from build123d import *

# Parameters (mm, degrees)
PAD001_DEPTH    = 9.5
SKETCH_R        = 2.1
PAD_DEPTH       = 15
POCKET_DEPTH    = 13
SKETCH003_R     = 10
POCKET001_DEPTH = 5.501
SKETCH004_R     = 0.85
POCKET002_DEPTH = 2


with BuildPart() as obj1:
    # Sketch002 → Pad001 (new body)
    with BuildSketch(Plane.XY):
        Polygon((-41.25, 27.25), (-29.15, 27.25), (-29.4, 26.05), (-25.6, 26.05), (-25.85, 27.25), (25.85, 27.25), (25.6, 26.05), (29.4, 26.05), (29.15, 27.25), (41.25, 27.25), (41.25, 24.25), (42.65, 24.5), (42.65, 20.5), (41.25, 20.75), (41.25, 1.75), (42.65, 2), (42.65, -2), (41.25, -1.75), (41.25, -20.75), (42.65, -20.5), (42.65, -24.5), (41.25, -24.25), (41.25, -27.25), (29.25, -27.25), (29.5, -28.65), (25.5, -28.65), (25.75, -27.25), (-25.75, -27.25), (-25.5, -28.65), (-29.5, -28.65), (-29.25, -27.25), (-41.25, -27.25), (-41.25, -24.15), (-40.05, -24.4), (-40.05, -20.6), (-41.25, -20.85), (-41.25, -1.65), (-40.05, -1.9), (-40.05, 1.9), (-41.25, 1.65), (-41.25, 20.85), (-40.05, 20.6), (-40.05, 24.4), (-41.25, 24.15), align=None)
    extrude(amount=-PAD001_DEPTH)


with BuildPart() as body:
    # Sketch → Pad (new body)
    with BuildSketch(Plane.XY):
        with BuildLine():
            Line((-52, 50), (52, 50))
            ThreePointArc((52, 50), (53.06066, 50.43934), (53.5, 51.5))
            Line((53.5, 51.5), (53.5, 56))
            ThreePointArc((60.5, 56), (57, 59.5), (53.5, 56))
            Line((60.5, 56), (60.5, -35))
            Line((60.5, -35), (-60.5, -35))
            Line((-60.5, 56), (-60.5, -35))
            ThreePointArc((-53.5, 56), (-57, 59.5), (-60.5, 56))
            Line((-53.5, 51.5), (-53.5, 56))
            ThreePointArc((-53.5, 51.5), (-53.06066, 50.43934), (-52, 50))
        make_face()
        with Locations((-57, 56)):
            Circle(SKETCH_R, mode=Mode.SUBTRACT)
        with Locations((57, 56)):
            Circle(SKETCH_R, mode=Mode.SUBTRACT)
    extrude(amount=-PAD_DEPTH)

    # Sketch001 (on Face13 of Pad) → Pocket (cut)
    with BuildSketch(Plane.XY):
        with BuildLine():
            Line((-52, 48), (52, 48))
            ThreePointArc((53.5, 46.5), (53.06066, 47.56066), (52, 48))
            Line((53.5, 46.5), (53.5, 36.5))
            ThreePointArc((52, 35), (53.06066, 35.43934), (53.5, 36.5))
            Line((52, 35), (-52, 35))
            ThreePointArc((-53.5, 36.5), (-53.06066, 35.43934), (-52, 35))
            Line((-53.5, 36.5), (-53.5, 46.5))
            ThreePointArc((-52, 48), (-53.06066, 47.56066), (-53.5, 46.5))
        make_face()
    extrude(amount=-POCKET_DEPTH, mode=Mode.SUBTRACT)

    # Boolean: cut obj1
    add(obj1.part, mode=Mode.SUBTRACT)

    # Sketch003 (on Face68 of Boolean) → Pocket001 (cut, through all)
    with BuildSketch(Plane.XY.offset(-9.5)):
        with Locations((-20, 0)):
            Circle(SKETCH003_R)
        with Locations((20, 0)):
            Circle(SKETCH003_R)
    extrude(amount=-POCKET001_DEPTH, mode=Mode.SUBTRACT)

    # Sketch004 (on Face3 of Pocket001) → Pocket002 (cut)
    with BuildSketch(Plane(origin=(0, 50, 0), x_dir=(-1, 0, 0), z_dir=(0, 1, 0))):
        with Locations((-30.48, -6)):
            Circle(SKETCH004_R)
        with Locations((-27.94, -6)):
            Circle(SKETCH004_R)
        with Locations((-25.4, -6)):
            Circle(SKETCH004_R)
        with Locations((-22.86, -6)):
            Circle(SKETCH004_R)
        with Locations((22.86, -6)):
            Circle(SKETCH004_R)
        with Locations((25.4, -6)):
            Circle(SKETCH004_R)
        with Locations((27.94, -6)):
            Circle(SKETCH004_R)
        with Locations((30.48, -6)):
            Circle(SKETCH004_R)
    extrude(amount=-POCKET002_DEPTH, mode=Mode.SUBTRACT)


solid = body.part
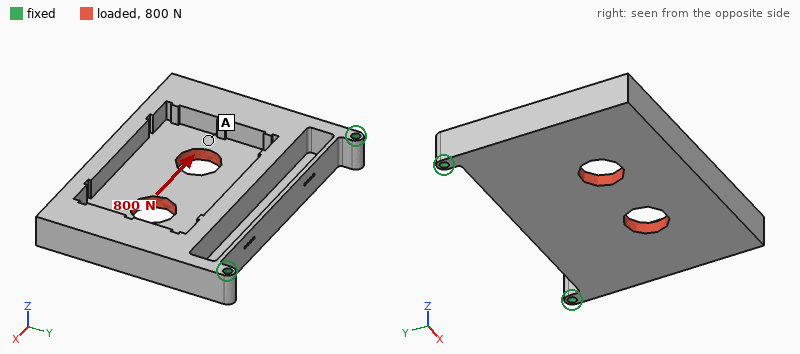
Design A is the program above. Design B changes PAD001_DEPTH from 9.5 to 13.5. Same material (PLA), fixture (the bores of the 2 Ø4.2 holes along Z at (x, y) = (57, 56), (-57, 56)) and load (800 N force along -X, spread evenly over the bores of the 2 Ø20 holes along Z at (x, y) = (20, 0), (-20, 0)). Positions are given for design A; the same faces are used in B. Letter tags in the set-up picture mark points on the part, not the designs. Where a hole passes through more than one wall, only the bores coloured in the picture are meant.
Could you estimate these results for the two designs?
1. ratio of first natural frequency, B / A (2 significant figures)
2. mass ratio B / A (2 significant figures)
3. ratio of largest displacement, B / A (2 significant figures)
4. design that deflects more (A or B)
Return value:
1.1
0.83
1.5
B
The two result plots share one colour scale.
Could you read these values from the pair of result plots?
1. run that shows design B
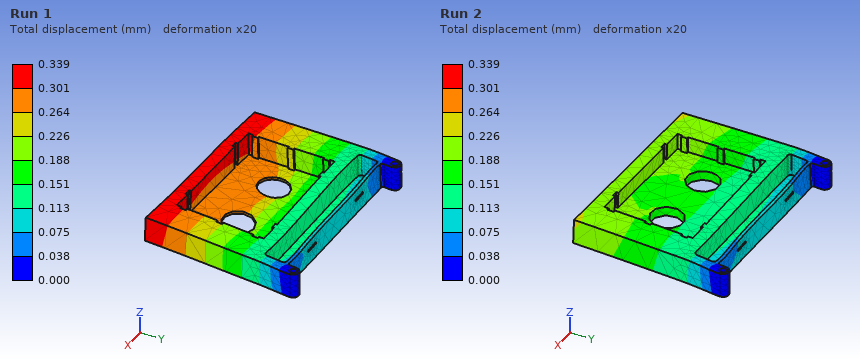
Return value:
Run 1
